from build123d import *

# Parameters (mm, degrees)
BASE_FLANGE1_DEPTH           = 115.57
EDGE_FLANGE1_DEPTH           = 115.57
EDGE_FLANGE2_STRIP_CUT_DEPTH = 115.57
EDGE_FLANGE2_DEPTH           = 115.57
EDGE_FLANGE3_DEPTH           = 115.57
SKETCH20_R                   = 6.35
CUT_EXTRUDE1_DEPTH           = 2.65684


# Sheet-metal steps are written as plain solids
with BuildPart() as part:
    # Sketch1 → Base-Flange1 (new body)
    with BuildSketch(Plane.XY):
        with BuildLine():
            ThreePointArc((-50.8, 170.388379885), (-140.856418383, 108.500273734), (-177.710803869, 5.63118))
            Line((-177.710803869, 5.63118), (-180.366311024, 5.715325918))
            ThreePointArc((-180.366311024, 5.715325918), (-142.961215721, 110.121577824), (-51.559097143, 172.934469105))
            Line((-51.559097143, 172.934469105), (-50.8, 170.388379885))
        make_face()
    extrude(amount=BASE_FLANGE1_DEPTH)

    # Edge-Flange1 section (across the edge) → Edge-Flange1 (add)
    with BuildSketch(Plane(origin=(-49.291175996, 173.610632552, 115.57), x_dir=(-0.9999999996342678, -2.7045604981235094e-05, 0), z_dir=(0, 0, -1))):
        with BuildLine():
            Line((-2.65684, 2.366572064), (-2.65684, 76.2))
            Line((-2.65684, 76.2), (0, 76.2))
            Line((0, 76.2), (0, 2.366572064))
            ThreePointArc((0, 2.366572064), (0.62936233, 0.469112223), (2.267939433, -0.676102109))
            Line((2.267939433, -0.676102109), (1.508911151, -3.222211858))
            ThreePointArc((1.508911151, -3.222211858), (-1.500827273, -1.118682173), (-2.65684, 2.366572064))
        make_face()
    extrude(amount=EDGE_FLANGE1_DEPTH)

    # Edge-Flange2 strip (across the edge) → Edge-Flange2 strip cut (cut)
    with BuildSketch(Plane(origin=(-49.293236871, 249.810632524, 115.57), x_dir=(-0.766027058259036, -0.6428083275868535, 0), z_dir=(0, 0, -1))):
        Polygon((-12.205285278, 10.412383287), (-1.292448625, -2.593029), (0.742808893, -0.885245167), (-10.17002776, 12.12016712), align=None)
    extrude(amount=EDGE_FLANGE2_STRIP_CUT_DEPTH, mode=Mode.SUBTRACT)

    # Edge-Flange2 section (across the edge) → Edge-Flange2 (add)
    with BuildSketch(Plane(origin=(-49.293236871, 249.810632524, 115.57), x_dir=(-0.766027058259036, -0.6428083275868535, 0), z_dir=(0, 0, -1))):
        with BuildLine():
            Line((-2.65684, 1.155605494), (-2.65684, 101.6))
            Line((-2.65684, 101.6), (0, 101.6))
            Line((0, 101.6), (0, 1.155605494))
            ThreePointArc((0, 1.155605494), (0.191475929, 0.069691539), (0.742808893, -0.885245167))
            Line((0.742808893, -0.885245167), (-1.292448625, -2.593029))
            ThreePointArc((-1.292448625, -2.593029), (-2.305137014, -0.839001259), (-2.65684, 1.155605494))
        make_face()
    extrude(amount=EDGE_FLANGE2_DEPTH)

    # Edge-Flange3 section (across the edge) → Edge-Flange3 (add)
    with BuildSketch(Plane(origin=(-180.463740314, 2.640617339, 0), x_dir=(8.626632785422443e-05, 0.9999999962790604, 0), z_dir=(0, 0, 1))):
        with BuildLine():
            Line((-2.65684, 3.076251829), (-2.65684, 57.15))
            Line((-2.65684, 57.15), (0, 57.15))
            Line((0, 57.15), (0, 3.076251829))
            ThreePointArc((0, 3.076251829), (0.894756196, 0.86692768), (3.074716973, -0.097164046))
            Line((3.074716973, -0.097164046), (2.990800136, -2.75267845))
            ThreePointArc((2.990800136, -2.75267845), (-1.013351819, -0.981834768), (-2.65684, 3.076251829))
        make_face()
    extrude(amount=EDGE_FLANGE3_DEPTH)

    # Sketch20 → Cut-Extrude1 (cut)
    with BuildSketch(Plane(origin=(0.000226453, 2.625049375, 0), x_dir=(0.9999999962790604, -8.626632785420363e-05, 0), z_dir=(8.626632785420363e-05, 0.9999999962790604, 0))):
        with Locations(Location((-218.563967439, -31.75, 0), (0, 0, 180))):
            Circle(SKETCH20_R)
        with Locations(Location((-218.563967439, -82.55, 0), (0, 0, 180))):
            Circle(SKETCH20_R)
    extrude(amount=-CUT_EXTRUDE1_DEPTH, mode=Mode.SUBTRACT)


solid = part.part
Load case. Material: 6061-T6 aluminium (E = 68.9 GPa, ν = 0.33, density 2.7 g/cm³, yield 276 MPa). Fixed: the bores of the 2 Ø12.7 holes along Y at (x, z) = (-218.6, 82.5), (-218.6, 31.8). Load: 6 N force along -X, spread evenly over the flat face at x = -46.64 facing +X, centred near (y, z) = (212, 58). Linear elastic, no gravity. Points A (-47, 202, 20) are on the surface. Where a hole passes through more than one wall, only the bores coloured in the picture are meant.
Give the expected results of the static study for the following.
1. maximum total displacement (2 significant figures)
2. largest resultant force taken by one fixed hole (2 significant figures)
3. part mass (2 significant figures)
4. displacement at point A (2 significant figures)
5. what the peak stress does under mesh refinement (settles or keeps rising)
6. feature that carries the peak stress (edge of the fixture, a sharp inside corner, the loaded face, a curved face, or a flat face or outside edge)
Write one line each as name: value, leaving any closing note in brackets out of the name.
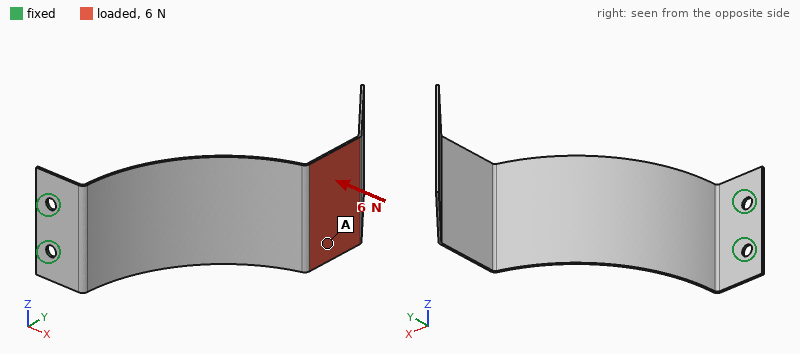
maximum total displacement: 4.1 mm
largest resultant force taken by one fixed hole: 3.9 N
part mass: 390 g
displacement at point A: 2.7 mm
what the peak stress does under mesh refinement: keeps rising
feature that carries the peak stress: edge of the fixture
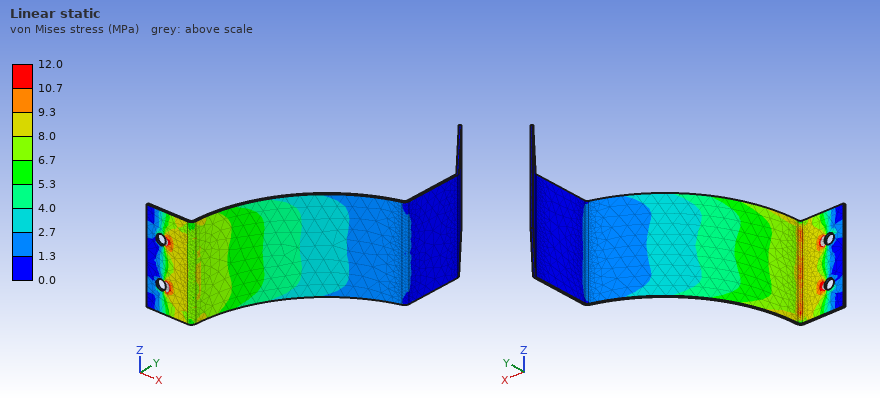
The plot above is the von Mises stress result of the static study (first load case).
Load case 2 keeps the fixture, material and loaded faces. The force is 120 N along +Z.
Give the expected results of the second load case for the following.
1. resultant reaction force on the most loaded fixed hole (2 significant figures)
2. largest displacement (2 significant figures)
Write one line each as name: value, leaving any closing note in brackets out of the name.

resultant reaction force on the most loaded fixed hole: 510 N
largest displacement: 4.6 mm
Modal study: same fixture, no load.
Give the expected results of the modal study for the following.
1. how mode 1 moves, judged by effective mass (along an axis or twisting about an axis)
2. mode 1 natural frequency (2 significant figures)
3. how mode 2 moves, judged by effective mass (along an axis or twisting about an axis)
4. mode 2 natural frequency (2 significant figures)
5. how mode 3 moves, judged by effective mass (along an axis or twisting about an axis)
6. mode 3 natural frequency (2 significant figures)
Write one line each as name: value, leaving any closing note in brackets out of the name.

how mode 1 moves, judged by effective mass: along X
mode 1 natural frequency: 13 Hz
how mode 2 moves, judged by effective mass: along Z
mode 2 natural frequency: 46 Hz
how mode 3 moves, judged by effective mass: along Y
mode 3 natural frequency: 66 Hz
